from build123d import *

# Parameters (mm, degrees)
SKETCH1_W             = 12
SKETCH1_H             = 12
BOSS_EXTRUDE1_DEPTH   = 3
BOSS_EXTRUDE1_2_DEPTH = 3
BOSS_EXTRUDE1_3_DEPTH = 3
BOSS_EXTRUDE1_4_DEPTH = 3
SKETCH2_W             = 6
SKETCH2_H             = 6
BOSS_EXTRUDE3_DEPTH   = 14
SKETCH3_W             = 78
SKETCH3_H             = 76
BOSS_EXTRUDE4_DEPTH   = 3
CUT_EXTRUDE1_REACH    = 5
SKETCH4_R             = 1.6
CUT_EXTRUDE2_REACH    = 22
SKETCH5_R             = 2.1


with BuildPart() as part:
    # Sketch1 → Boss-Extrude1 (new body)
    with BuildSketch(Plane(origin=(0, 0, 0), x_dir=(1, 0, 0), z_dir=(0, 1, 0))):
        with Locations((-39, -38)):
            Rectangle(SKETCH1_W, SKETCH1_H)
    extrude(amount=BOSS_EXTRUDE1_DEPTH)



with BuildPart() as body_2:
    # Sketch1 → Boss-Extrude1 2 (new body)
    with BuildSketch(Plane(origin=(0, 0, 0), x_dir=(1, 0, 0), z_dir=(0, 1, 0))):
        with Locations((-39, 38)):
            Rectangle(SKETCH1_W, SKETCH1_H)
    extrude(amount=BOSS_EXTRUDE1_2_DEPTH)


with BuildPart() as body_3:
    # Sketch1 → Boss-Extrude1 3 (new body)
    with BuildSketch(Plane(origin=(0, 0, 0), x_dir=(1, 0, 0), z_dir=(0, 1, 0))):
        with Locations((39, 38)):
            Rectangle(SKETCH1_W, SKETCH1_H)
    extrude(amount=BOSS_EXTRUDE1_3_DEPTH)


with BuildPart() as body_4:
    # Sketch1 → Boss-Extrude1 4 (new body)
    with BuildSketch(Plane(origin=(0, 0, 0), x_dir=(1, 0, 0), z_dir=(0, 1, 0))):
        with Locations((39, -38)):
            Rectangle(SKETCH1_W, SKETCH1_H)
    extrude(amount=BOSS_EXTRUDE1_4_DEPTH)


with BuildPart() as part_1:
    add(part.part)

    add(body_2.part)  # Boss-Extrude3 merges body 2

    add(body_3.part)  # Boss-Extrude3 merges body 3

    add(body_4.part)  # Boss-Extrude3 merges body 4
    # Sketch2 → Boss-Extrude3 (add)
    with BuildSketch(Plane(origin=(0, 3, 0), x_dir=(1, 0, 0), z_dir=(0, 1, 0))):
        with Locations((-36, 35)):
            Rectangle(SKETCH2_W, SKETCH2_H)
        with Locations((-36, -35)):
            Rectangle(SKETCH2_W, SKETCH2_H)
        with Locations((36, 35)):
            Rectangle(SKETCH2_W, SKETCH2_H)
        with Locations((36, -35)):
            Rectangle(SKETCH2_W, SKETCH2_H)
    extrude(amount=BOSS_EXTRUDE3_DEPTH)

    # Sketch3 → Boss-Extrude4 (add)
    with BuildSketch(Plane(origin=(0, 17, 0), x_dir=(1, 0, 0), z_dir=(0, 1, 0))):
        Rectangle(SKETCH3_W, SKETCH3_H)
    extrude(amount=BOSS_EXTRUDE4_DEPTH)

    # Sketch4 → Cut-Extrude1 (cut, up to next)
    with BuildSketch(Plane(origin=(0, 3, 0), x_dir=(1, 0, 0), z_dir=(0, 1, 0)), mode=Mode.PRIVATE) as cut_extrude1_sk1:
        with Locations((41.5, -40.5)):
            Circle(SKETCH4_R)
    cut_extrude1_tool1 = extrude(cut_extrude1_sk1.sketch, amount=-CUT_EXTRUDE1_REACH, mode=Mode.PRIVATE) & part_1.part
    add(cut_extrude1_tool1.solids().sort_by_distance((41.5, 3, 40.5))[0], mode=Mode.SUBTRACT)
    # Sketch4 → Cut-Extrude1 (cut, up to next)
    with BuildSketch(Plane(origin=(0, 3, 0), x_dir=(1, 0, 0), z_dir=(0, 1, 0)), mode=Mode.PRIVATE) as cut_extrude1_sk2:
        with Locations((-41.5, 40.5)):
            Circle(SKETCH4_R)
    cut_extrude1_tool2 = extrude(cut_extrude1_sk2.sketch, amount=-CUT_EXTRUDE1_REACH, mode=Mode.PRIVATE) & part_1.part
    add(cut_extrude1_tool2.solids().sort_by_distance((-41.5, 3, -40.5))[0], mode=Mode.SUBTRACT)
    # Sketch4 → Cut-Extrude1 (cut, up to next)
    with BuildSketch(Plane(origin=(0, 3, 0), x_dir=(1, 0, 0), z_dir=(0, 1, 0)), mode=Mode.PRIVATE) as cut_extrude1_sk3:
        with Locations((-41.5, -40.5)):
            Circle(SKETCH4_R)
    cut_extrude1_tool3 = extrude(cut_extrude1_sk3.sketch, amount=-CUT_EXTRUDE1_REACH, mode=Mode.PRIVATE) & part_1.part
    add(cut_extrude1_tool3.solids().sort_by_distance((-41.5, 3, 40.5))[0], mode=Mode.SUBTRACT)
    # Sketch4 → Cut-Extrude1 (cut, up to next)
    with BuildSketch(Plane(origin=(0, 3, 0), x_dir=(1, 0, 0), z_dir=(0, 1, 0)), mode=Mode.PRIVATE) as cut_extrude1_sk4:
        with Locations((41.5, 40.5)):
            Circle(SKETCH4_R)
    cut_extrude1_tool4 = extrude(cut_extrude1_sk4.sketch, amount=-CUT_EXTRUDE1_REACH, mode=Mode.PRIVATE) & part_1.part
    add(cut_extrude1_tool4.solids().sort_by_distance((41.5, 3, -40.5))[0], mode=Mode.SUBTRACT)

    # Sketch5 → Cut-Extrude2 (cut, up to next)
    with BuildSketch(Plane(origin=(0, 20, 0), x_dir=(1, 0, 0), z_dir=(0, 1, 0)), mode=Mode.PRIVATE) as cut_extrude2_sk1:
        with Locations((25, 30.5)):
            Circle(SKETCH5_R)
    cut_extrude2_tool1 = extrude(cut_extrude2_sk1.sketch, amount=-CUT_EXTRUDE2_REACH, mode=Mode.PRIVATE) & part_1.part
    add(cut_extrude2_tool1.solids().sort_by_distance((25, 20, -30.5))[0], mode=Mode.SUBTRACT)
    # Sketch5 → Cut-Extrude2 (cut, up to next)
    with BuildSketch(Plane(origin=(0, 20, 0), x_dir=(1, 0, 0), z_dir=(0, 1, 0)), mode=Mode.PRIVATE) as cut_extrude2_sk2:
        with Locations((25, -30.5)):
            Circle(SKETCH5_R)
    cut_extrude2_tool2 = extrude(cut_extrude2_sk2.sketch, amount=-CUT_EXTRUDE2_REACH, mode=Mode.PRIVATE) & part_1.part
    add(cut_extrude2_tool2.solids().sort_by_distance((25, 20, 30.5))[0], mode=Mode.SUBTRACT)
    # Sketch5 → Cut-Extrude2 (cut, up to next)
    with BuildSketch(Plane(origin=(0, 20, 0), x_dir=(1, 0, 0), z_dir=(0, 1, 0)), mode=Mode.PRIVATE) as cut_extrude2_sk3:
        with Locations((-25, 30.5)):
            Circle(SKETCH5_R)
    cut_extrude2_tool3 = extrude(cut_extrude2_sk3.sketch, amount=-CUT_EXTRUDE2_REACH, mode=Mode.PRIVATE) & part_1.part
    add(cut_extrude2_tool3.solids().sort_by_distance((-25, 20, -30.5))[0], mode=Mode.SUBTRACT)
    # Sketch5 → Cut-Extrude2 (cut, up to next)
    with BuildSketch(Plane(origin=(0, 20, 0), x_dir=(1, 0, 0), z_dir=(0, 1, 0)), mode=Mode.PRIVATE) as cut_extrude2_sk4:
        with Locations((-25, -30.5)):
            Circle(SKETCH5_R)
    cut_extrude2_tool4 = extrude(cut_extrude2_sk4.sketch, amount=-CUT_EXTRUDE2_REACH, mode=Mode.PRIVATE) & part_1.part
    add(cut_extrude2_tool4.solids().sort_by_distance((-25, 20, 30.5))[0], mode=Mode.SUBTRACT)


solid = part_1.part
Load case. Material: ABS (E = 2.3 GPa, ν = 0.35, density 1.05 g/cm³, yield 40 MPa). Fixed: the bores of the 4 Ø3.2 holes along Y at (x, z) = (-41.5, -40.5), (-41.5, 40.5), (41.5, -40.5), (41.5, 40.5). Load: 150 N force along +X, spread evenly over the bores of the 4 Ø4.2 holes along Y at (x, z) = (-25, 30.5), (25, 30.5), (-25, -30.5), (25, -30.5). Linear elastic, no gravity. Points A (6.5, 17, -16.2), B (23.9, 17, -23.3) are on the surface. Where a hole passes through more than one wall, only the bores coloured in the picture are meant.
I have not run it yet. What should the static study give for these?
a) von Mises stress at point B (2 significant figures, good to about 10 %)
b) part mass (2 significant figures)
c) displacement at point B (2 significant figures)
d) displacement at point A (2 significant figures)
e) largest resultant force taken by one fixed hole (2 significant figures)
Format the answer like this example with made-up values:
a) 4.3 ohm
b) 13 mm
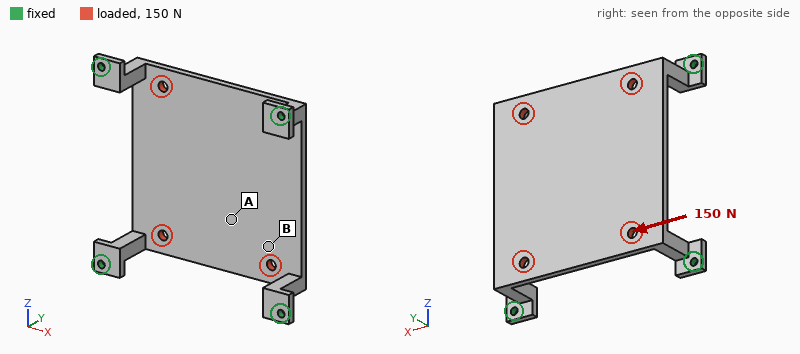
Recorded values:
a) 4.1 MPa
b) 22 g
c) 0.60 mm
d) 0.59 mm
e) 38 N
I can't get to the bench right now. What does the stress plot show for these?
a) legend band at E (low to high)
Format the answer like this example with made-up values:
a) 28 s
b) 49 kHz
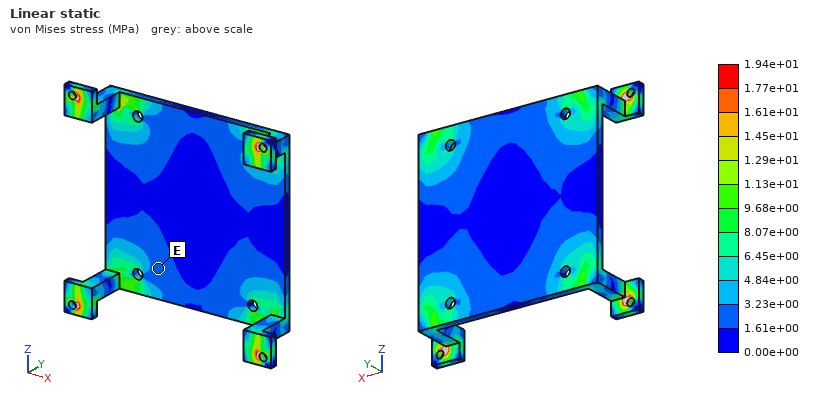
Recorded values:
a) 1.61e+00 to 3.23e+00 MPa
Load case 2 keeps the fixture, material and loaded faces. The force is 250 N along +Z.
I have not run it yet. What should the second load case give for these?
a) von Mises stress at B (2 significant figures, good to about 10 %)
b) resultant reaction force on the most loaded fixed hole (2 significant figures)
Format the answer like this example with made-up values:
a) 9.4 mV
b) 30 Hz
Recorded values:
a) 4.4 MPa
b) 64 N
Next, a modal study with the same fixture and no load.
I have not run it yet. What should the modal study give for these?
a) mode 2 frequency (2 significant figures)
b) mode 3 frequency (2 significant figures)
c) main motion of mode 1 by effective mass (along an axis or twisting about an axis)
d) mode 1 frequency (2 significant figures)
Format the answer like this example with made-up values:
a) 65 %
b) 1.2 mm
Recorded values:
a) 560 Hz
b) 570 Hz
c) along Y
d) 540 Hz
